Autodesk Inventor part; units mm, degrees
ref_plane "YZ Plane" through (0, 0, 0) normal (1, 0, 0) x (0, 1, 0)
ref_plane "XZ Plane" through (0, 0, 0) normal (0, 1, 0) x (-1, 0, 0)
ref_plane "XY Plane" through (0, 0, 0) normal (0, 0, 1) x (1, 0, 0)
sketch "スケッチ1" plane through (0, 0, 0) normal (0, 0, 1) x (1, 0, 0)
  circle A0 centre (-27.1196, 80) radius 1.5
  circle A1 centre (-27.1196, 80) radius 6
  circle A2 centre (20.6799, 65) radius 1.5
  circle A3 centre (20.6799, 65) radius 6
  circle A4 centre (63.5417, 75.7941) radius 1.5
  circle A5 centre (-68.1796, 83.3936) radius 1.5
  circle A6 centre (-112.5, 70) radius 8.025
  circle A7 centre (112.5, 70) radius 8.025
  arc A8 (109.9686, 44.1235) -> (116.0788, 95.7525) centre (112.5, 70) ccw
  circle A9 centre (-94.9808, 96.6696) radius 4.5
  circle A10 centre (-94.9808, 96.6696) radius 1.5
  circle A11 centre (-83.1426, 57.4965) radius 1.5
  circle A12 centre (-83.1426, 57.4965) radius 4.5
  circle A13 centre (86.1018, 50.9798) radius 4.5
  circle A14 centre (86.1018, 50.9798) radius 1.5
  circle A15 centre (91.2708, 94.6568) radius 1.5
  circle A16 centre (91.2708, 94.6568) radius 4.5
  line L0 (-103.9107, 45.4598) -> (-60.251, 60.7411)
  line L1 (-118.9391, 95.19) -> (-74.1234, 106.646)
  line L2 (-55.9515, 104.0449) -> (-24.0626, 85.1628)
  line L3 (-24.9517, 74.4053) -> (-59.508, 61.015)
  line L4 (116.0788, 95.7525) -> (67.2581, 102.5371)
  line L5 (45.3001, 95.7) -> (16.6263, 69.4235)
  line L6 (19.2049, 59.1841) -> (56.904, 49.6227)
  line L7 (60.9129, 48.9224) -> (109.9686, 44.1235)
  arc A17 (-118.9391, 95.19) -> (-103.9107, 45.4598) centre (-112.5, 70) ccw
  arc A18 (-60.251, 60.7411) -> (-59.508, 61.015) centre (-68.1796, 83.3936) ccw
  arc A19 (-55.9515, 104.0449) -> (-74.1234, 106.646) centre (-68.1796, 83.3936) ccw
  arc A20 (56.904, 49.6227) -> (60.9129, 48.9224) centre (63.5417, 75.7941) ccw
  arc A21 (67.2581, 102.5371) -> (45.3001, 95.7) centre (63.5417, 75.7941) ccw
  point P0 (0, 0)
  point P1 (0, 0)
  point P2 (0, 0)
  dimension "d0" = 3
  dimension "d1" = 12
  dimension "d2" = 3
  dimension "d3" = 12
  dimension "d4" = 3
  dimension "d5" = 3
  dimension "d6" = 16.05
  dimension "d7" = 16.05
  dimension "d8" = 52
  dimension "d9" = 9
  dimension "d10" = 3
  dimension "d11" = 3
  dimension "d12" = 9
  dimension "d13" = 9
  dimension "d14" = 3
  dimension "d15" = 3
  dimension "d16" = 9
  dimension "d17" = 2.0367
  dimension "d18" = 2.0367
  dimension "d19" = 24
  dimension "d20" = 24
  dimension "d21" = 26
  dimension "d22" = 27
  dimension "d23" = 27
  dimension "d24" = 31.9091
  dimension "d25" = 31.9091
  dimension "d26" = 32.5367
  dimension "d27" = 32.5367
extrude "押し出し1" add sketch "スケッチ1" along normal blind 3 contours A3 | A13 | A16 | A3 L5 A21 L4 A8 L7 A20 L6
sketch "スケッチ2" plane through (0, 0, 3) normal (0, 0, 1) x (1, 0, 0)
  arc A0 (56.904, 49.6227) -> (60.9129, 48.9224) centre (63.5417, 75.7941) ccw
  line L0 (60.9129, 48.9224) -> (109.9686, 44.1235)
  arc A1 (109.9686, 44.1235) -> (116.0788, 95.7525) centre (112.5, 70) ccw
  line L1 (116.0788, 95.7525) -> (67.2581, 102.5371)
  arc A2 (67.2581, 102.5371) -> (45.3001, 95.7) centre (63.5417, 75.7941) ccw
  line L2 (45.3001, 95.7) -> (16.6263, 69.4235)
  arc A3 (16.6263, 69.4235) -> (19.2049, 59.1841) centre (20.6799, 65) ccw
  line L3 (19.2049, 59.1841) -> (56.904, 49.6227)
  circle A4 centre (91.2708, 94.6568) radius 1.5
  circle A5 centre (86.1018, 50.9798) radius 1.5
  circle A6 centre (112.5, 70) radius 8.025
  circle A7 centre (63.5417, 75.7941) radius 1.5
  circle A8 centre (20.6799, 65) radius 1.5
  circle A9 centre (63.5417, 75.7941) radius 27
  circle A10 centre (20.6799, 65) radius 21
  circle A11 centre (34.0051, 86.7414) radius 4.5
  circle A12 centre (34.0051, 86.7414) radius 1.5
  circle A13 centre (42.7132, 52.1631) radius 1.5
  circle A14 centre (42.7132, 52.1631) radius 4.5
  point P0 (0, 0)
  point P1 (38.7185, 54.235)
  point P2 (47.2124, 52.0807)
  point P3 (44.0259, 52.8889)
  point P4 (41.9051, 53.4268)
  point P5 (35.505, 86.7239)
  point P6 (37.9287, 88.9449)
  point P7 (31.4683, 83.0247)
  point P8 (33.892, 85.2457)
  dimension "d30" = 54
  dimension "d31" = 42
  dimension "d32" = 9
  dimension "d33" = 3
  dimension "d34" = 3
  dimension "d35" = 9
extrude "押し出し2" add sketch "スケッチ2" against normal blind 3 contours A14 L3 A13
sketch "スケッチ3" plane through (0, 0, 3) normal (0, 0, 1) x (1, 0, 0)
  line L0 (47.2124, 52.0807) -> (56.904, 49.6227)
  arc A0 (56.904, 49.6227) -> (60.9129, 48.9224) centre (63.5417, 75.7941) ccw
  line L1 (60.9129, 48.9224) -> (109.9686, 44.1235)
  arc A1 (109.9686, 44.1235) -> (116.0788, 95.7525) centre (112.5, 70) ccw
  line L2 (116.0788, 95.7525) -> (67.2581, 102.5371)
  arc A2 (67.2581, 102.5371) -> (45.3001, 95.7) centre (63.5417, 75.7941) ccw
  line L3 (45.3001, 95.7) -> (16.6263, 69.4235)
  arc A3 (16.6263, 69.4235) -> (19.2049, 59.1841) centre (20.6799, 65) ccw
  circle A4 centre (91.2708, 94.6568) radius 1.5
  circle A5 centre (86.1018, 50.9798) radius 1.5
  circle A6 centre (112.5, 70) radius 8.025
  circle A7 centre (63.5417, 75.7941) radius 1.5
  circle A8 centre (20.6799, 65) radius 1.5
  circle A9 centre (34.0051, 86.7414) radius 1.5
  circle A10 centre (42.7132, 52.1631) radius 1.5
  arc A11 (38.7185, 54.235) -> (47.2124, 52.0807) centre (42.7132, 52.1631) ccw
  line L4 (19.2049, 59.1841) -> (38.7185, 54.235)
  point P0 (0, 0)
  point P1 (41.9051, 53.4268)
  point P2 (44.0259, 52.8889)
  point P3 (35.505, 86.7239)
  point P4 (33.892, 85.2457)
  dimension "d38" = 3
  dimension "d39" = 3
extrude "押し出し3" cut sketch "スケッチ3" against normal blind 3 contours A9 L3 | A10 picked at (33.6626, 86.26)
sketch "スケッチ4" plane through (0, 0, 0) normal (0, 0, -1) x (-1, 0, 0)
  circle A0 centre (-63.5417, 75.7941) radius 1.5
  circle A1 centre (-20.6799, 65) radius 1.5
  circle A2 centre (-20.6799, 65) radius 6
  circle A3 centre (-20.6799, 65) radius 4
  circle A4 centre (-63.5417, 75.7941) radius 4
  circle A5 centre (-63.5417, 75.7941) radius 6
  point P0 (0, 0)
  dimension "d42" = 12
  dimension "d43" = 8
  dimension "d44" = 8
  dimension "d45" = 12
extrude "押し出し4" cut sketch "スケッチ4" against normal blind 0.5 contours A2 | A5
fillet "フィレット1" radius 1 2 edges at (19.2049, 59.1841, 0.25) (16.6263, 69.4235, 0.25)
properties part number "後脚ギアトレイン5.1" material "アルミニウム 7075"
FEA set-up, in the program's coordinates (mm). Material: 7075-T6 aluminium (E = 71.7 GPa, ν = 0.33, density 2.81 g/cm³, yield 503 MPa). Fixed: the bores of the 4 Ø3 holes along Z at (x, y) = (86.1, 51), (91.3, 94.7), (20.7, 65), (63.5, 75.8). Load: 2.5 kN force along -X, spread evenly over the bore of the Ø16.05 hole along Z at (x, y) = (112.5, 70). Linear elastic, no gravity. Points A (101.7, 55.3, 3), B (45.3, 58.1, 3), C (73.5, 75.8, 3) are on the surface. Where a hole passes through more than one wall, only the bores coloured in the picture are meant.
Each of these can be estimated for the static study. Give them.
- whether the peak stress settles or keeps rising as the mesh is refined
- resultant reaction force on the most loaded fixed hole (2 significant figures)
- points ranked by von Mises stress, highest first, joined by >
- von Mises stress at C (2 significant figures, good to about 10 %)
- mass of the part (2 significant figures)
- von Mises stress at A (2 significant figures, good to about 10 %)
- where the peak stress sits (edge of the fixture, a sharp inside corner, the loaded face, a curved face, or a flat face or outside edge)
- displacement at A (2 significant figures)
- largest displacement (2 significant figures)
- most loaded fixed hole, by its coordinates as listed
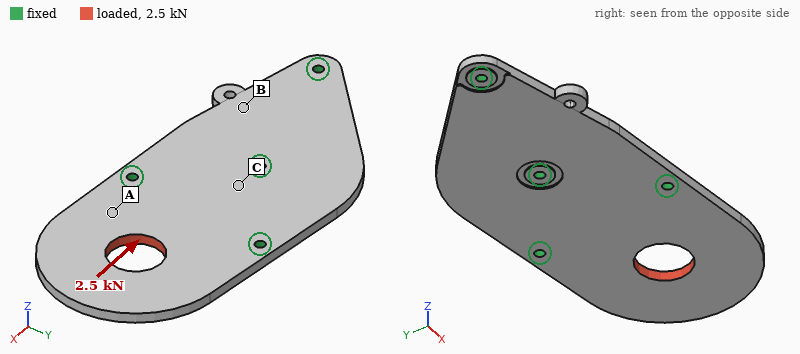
keeps rising
1.2 kN
A > C > B
12 MPa
43 g
22 MPa
edge of the fixture
6.2 µm
14 µm
(86.1, 51)
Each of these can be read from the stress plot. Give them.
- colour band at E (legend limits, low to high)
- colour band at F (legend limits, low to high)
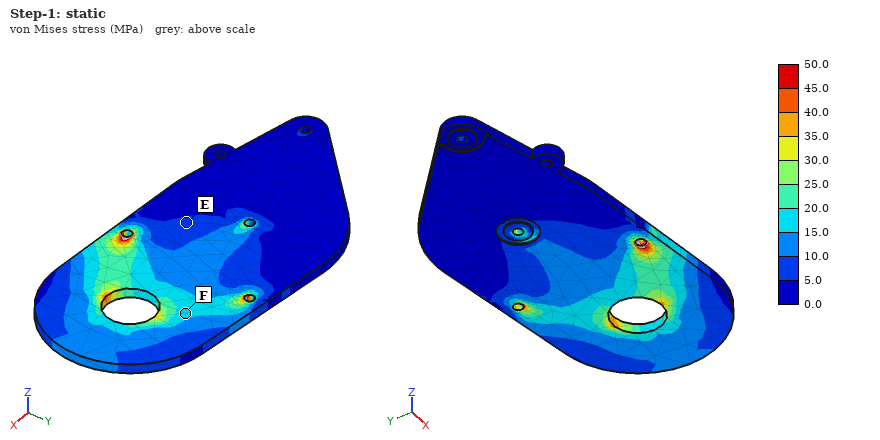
5.0 to 10.0 MPa
15.0 to 20.0 MPa
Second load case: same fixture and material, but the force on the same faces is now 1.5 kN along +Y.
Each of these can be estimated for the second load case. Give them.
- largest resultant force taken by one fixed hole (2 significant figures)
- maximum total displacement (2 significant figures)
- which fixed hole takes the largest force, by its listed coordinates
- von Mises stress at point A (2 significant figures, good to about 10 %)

1.1 kN
24 µm
(91.3, 94.7)
17 MPa
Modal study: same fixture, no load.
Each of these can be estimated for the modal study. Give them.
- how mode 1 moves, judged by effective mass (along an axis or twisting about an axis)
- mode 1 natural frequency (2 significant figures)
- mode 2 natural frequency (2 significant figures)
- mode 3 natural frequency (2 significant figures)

along Z
1100 Hz
3000 Hz
3800 Hz
